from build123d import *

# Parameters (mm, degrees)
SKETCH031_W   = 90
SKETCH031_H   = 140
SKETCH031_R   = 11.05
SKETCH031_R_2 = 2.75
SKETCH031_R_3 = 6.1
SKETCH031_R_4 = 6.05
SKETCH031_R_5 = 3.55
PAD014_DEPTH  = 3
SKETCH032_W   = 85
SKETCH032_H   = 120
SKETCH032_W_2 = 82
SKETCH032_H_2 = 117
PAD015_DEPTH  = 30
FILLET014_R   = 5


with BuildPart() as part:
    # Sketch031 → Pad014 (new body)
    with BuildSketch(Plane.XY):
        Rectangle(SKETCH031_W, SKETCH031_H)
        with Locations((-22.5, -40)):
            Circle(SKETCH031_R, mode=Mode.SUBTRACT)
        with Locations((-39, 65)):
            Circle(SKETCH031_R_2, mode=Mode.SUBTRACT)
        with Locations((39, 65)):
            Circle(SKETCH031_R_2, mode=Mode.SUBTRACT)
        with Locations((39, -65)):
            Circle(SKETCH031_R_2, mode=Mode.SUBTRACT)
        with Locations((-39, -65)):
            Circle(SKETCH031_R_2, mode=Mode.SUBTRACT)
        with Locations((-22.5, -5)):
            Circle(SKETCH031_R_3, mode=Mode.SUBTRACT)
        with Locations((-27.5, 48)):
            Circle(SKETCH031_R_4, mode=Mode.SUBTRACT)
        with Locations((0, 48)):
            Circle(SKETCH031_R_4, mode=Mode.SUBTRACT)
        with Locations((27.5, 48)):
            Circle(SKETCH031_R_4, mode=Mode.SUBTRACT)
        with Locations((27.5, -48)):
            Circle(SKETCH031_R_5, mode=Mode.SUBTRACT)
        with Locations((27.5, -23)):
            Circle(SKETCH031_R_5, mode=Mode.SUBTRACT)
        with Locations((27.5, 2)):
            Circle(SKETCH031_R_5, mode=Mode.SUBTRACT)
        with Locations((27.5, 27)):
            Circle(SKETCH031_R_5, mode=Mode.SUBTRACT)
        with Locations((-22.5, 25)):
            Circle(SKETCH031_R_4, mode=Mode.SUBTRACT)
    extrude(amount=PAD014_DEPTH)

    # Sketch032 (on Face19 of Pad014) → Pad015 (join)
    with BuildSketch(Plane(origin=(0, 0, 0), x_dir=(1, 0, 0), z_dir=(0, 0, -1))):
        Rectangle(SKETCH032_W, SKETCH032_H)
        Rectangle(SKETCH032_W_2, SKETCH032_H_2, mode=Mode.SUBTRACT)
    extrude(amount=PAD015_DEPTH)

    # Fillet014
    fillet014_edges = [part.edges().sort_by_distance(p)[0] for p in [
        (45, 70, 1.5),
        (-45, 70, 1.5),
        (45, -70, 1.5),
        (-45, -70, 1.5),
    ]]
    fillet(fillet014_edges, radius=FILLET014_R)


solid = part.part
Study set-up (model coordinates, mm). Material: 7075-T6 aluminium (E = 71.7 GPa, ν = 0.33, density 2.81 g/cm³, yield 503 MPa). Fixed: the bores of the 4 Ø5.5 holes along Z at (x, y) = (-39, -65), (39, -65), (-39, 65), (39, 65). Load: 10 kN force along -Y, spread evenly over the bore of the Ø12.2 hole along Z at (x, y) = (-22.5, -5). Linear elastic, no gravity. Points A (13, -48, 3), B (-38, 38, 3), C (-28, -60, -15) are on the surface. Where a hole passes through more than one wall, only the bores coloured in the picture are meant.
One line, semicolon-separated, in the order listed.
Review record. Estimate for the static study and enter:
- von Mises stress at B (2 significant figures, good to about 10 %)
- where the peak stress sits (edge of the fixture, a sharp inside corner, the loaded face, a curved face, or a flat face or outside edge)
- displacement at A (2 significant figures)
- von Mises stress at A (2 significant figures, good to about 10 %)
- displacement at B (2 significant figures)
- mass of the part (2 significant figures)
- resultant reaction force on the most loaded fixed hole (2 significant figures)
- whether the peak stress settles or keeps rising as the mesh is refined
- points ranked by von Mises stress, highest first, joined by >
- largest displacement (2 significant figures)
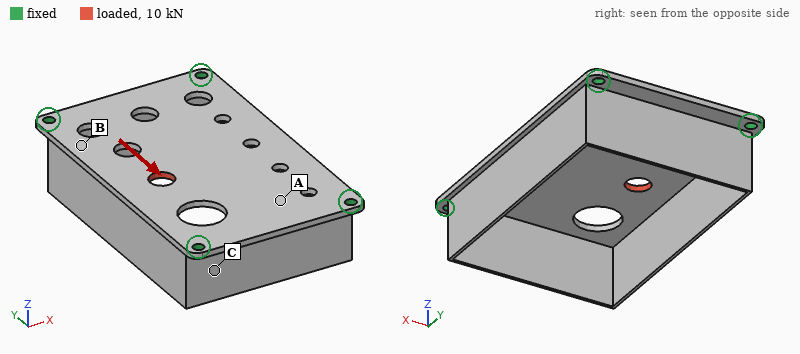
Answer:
55 MPa; edge of the fixture; 21 µm; 28 MPa; 25 µm; 150 g; 3.2 kN; keeps rising; B > A > C; 58 µm
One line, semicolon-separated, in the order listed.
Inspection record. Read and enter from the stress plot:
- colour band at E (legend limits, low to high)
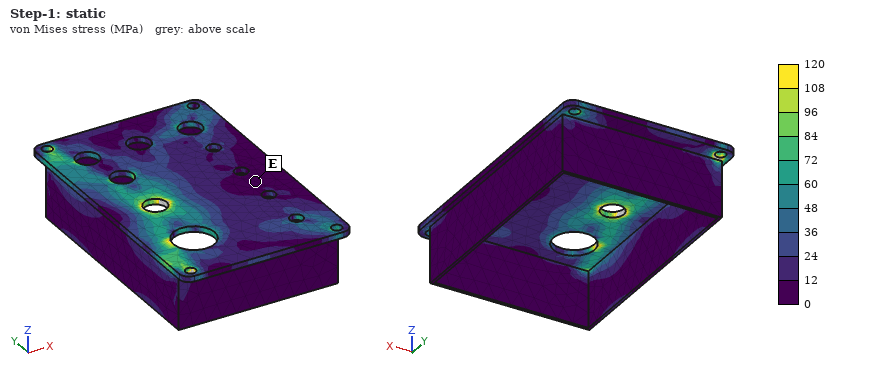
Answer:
0 to 12 MPa
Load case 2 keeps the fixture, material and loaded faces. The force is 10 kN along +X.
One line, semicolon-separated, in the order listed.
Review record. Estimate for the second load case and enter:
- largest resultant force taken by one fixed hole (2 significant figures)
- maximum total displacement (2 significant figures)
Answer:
3.6 kN; 0.11 mm
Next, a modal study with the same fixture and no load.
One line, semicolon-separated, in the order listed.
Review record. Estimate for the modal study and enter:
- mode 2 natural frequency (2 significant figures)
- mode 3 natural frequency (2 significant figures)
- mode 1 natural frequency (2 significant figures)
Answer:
1500 Hz; 1700 Hz; 1300 Hz
